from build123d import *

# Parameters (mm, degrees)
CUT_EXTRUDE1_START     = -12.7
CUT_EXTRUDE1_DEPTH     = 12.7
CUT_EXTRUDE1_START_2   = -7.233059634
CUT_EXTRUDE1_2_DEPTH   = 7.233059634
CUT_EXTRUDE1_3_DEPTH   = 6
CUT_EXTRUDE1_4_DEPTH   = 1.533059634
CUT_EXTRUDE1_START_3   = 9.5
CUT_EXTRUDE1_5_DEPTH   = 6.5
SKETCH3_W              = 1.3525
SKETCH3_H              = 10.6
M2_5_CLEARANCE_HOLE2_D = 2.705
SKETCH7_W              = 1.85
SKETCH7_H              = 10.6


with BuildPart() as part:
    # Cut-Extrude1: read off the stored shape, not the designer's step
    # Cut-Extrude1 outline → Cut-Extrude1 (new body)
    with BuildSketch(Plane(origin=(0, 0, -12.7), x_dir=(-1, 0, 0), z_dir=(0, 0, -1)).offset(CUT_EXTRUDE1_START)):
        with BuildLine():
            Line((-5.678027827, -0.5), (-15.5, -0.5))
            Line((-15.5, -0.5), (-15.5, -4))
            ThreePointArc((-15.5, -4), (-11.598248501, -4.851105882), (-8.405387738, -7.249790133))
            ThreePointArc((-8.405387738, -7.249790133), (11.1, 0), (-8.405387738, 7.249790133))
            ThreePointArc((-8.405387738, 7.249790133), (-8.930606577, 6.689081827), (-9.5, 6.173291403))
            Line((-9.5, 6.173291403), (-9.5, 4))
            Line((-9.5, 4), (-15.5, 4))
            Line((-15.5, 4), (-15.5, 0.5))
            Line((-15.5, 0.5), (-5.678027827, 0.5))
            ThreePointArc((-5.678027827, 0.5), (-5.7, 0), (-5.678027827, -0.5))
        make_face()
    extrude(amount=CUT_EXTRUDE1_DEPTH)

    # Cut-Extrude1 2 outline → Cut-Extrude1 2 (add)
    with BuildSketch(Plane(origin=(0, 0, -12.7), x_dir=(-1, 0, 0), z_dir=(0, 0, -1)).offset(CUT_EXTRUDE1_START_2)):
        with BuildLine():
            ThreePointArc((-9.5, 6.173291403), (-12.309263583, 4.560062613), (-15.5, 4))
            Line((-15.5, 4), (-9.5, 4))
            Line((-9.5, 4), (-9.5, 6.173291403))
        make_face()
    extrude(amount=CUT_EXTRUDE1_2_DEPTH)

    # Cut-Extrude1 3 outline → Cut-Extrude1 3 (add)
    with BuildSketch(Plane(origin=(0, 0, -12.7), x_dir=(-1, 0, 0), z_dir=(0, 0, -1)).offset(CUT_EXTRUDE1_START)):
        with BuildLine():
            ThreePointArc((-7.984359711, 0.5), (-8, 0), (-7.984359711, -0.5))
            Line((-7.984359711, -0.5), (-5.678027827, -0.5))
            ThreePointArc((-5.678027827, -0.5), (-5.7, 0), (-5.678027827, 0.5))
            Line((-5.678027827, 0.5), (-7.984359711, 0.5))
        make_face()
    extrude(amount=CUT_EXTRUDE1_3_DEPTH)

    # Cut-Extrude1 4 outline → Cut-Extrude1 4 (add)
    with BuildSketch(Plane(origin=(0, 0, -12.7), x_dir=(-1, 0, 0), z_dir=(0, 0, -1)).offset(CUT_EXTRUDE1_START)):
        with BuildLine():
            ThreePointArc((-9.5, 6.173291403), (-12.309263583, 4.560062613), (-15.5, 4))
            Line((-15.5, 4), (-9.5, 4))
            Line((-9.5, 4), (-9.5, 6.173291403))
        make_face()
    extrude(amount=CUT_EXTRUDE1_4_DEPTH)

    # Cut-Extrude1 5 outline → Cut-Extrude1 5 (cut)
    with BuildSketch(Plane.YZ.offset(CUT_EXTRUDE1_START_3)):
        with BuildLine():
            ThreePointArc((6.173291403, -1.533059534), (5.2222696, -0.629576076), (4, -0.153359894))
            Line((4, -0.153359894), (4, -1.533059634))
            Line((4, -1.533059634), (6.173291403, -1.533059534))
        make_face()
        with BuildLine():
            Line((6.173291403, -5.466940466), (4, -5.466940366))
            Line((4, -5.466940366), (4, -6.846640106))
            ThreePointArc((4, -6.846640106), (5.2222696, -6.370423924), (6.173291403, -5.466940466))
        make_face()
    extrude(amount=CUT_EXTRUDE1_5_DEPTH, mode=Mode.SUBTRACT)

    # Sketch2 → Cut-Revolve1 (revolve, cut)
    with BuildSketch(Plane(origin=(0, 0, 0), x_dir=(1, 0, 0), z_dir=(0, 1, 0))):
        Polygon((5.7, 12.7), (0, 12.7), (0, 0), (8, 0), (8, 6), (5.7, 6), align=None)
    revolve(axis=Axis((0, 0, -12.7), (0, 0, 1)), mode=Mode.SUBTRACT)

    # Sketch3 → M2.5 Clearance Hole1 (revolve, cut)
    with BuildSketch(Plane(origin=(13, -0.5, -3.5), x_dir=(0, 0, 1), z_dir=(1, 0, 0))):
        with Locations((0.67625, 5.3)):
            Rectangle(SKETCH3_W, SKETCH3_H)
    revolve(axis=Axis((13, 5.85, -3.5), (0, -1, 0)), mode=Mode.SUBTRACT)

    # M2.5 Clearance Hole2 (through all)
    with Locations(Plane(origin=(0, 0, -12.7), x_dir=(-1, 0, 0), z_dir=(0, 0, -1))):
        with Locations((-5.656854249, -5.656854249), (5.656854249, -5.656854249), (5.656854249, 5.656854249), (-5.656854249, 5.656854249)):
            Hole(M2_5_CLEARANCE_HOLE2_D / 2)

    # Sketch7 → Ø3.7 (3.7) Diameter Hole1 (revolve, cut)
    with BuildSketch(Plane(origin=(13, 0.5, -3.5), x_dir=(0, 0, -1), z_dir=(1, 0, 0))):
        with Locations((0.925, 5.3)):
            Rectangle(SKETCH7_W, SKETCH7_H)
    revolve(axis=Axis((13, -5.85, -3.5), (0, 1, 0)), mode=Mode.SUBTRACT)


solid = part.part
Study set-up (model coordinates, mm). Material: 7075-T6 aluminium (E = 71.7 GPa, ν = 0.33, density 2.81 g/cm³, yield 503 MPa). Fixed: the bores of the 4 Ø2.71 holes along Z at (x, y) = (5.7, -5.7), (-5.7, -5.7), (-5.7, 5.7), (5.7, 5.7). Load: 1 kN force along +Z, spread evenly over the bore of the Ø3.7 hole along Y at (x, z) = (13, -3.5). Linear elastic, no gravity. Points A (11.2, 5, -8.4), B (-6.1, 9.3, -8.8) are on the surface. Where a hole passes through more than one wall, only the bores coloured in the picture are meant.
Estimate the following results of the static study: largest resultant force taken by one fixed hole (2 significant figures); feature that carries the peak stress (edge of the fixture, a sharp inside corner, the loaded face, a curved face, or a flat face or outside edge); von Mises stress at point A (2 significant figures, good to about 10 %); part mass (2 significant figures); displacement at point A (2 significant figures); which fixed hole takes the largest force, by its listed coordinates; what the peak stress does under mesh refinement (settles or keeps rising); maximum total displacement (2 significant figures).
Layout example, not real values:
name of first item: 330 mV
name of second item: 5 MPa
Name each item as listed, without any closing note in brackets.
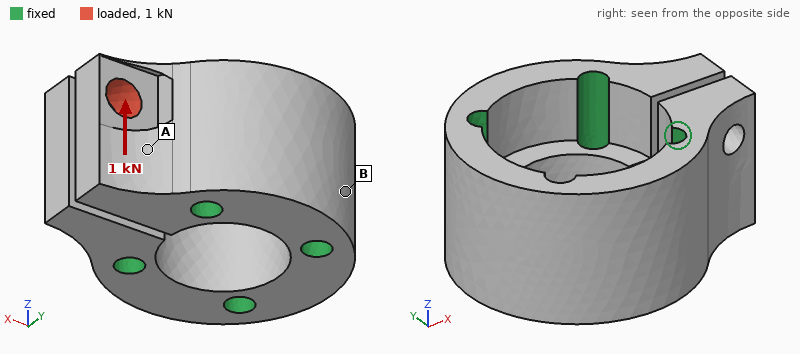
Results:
largest resultant force taken by one fixed hole: 1.0 kN
feature that carries the peak stress: edge of the fixture
von Mises stress at point A: 71 MPa
part mass: 8.9 g
displacement at point A: 5.7 µm
which fixed hole takes the largest force, by its listed coordinates: (5.7, 5.7)
what the peak stress does under mesh refinement: keeps rising
maximum total displacement: 24 µm
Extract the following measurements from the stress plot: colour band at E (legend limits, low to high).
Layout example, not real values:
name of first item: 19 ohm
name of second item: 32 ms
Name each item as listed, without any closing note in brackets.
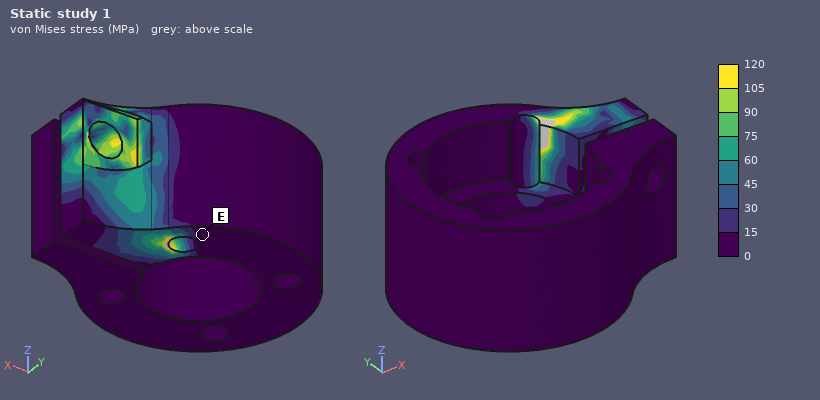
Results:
colour band at E: 0 to 15 MPa
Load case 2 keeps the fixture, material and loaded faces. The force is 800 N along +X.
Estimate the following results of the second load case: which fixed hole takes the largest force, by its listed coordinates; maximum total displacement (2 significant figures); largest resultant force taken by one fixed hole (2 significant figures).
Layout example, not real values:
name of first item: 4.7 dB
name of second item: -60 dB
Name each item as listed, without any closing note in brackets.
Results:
which fixed hole takes the largest force, by its listed coordinates: (5.7, 5.7)
maximum total displacement: 27 µm
largest resultant force taken by one fixed hole: 860 N
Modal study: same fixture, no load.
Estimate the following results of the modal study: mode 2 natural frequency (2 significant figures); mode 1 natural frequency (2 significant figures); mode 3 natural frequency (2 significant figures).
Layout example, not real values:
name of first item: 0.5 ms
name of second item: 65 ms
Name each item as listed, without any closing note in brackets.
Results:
mode 2 natural frequency: 34 kHz
mode 1 natural frequency: 34 kHz
mode 3 natural frequency: 50 kHz
